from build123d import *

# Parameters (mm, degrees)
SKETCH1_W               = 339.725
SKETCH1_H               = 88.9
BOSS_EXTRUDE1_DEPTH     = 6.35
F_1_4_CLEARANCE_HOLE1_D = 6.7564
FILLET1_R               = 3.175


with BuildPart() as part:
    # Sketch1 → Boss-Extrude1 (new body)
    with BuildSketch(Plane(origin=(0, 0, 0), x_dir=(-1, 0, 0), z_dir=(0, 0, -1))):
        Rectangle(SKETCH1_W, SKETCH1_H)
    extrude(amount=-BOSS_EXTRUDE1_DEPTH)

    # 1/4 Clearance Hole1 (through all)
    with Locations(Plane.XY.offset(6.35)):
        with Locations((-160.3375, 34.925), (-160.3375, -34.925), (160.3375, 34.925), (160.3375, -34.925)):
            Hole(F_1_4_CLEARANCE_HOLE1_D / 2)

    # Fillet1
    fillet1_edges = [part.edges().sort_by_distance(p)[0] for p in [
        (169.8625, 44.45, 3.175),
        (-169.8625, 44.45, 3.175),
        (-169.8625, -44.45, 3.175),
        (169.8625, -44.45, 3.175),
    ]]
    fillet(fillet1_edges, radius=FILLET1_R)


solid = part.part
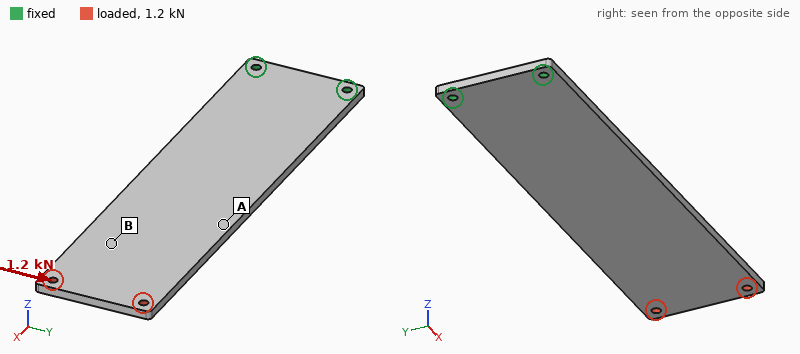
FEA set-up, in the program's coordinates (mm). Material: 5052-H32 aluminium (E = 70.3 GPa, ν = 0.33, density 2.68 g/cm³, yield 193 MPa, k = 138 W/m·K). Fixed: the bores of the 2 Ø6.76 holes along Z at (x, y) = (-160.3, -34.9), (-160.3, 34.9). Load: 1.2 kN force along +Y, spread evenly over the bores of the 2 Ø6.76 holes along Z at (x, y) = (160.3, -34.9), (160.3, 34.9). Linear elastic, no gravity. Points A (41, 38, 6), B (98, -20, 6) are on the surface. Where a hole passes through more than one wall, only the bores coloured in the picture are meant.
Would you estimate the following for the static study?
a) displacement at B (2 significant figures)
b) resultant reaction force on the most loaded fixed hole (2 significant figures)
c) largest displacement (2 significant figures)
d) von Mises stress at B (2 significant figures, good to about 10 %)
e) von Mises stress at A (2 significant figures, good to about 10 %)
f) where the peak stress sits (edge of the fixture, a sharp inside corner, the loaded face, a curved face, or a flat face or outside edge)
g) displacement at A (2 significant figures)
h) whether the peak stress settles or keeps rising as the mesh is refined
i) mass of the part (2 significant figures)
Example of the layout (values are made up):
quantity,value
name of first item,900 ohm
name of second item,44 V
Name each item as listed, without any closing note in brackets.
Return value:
quantity,value
displacement at B,0.40 mm
resultant reaction force on the most loaded fixed hole,5.4 kN
largest displacement,0.58 mm
von Mises stress at B,5.9 MPa
von Mises stress at A,15 MPa
where the peak stress sits,edge of the fixture
displacement at A,0.28 mm
whether the peak stress settles or keeps rising as the mesh is refined,keeps rising
mass of the part,510 g
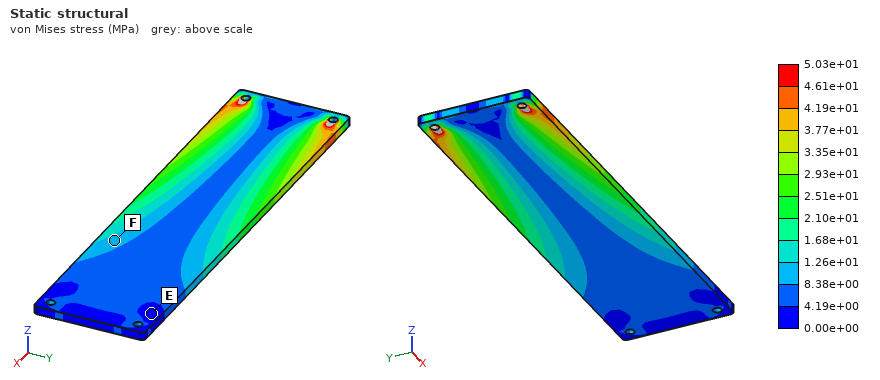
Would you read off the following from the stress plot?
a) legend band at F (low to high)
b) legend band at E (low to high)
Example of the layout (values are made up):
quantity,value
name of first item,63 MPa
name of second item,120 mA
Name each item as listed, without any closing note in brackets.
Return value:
quantity,value
legend band at F,8.38e+00 to 1.26e+01 MPa
legend band at E,0.00e+00 to 4.19e+00 MPa
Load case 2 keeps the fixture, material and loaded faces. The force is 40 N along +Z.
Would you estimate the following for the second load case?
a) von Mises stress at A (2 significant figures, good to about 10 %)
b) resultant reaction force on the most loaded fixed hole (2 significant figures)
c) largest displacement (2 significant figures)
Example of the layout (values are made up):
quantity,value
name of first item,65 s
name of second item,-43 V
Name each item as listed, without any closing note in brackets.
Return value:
quantity,value
von Mises stress at A,8.0 MPa
resultant reaction force on the most loaded fixed hole,20 N
largest displacement,3.6 mm
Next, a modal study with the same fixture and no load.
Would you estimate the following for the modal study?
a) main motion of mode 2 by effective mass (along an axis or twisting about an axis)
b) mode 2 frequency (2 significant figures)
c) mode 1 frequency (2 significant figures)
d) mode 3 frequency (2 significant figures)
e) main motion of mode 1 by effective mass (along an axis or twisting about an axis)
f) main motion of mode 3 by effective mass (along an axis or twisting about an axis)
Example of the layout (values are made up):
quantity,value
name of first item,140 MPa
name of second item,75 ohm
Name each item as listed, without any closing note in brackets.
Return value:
quantity,value
main motion of mode 2 by effective mass,along Z
mode 2 frequency,300 Hz
mode 1 frequency,47 Hz
mode 3 frequency,360 Hz
main motion of mode 1 by effective mass,along Z
main motion of mode 3 by effective mass,twisting about X
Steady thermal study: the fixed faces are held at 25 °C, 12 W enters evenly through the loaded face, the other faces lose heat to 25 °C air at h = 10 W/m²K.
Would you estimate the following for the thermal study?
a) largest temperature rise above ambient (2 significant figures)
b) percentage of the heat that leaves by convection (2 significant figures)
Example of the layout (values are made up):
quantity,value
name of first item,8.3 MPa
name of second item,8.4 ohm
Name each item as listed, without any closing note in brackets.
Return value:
quantity,value
largest temperature rise above ambient,30 K
percentage of the heat that leaves by convection,64 %
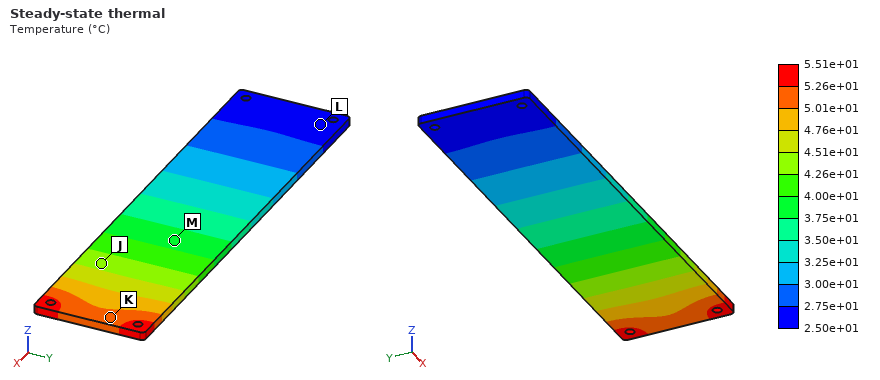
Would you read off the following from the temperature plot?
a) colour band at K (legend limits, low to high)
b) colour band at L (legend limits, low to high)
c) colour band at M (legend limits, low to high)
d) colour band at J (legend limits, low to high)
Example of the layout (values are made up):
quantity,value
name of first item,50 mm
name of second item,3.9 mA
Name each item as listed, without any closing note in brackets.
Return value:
quantity,value
colour band at K,5.01e+01 to 5.26e+01 °C
colour band at L,2.50e+01 to 2.75e+01 °C
colour band at M,3.75e+01 to 4.00e+01 °C
colour band at J,4.26e+01 to 4.51e+01 °C
